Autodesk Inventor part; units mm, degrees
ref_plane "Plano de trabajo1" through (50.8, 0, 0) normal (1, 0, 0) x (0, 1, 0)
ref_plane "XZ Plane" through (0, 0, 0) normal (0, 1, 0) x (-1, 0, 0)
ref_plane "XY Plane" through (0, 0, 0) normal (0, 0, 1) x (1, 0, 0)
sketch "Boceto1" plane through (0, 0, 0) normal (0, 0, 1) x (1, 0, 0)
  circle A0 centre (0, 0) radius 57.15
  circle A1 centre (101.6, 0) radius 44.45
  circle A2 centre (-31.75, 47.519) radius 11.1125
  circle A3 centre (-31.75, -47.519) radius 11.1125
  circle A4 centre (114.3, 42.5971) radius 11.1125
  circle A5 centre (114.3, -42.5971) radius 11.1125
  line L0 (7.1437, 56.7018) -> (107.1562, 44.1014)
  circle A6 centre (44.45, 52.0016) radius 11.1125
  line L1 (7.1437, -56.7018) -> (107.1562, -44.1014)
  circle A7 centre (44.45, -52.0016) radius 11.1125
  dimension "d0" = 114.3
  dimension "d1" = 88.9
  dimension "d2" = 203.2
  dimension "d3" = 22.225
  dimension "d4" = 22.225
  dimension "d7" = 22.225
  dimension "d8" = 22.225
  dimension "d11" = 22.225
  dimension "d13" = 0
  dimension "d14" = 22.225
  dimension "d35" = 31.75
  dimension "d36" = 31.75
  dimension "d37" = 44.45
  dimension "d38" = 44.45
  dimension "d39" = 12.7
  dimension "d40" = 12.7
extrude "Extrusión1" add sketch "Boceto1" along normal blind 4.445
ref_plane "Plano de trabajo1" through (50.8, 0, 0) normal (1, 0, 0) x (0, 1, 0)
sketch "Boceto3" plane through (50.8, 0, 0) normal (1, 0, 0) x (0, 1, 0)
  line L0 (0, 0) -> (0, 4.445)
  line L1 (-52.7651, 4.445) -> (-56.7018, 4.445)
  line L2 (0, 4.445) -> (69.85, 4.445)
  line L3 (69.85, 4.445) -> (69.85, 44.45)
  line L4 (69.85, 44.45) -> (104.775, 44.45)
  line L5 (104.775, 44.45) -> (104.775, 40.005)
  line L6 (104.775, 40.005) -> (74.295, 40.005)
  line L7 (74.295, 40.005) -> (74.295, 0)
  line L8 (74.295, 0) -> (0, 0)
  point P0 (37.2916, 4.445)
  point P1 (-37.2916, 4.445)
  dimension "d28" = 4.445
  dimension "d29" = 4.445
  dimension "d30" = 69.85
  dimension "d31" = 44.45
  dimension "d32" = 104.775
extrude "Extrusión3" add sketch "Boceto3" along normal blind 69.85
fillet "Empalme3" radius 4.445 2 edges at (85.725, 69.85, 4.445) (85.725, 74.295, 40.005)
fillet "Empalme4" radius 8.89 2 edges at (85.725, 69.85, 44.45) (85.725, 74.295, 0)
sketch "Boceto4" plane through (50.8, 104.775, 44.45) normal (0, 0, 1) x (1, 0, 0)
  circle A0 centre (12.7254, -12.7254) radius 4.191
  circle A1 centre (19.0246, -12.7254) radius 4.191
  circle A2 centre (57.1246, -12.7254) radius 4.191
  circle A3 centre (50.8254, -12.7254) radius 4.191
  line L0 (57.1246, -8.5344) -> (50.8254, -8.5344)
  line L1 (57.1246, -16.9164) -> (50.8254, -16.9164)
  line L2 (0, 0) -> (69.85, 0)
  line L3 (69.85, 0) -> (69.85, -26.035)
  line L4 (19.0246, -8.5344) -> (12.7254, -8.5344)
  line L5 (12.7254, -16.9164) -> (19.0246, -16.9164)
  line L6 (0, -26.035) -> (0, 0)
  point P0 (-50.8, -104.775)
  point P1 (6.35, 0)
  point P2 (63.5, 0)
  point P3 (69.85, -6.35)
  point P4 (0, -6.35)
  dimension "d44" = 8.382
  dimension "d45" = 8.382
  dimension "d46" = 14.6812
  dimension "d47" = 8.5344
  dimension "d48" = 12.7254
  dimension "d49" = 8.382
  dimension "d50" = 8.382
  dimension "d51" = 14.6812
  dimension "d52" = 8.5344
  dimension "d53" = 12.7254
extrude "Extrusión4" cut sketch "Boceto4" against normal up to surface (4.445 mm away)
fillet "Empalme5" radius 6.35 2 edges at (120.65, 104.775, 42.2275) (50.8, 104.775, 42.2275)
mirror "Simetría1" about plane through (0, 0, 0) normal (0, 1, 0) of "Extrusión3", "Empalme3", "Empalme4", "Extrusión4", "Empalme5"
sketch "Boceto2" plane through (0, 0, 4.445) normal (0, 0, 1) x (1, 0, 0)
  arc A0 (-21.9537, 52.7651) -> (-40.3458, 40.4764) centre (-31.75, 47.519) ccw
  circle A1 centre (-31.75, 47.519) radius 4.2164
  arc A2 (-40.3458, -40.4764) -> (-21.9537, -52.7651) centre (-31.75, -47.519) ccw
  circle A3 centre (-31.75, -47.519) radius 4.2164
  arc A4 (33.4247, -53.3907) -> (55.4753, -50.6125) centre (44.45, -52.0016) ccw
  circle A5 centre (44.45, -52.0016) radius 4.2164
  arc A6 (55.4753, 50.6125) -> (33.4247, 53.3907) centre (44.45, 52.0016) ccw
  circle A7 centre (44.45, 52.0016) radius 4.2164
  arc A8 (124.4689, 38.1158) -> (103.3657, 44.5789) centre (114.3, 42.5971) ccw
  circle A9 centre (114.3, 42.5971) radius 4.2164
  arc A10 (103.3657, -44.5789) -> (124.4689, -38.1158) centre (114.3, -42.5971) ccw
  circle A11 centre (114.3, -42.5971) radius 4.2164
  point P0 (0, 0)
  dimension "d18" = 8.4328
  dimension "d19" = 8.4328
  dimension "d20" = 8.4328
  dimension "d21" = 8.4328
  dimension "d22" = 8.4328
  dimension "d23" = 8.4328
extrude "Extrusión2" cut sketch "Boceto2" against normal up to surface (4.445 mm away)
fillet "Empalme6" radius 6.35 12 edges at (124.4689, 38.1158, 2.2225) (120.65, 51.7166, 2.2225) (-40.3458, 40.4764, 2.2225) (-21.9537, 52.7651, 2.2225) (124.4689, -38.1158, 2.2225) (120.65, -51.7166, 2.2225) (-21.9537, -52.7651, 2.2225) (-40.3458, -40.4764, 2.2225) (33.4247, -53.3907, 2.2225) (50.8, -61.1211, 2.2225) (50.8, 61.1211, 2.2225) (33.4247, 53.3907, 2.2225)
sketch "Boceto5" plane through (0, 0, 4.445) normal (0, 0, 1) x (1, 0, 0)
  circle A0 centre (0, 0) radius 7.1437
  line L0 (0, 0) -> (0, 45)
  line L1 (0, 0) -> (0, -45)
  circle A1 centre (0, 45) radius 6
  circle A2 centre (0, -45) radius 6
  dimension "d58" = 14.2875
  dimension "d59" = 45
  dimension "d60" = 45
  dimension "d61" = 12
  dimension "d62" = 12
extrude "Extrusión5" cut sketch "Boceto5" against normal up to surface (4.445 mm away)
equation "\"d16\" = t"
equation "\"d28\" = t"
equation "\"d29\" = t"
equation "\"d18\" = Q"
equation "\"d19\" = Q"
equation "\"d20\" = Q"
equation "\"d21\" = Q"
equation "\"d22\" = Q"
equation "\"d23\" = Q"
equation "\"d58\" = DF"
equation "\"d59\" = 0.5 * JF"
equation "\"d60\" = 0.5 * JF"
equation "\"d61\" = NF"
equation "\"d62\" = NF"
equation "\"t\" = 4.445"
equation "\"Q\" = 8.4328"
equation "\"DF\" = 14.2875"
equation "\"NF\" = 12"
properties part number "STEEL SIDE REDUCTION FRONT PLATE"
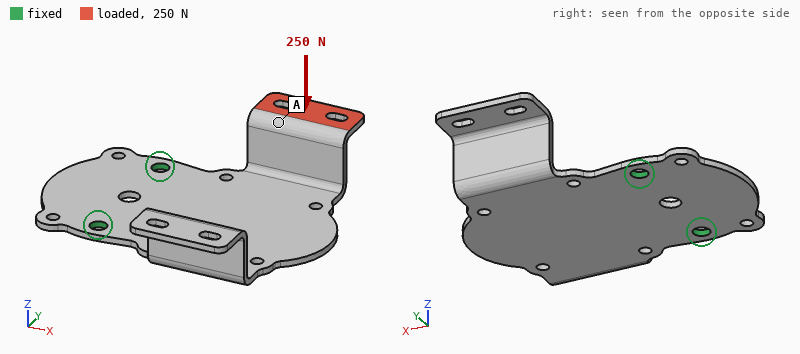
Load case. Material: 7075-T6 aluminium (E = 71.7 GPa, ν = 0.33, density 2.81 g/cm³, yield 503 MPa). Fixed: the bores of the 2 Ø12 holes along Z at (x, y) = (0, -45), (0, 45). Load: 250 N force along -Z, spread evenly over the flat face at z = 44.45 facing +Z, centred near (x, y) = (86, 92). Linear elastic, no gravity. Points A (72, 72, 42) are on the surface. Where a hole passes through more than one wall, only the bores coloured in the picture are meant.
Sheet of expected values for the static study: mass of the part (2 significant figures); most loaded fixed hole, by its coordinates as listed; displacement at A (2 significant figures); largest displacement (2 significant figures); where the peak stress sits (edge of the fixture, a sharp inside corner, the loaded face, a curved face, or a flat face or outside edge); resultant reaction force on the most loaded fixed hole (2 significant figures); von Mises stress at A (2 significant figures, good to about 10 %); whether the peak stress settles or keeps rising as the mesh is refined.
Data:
390 g
(0, 45)
1.8 mm
3.4 mm
edge of the fixture
370 N
14 MPa
keeps rising
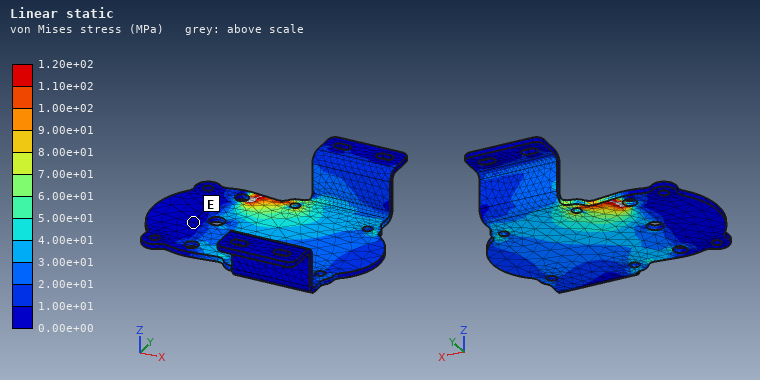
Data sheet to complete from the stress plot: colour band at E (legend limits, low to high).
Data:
0.00e+00 to 1.00e+01 MPa
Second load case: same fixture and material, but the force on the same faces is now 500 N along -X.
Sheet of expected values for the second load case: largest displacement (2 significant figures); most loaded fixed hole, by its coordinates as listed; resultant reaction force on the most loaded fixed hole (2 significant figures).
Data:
3.4 mm
(0, 45)
750 N
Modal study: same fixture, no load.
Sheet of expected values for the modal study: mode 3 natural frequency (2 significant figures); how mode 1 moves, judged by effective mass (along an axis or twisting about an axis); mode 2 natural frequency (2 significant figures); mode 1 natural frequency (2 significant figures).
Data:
410 Hz
along Z
220 Hz
140 Hz
